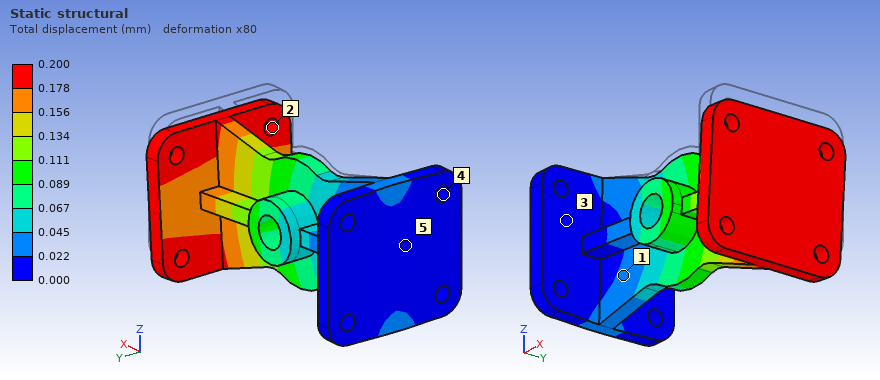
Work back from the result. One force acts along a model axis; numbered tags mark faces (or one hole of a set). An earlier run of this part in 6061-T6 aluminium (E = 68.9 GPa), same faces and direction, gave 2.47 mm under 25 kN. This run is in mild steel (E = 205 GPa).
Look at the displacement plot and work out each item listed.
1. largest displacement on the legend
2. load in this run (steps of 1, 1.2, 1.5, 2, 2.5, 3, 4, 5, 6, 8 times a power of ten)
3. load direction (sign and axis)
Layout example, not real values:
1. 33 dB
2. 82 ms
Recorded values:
1. 0.200 mm
2. 6 kN
3. -Z
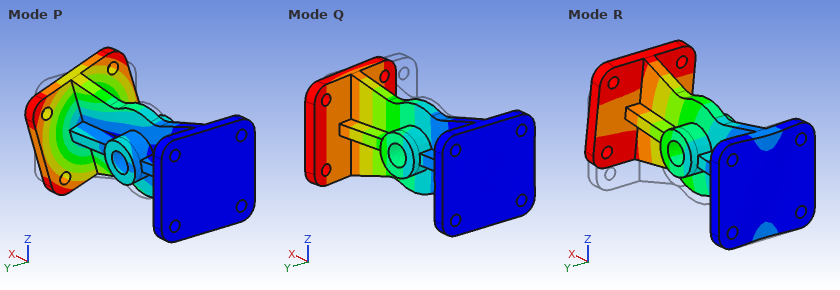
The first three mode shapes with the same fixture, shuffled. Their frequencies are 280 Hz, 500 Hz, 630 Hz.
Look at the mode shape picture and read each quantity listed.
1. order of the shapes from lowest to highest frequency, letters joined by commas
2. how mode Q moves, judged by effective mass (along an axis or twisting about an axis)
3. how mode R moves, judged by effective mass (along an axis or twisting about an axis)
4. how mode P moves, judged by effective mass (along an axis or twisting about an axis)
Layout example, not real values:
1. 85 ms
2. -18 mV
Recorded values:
1. Q, R, P
2. along Y
3. along Z
4. twisting about X
